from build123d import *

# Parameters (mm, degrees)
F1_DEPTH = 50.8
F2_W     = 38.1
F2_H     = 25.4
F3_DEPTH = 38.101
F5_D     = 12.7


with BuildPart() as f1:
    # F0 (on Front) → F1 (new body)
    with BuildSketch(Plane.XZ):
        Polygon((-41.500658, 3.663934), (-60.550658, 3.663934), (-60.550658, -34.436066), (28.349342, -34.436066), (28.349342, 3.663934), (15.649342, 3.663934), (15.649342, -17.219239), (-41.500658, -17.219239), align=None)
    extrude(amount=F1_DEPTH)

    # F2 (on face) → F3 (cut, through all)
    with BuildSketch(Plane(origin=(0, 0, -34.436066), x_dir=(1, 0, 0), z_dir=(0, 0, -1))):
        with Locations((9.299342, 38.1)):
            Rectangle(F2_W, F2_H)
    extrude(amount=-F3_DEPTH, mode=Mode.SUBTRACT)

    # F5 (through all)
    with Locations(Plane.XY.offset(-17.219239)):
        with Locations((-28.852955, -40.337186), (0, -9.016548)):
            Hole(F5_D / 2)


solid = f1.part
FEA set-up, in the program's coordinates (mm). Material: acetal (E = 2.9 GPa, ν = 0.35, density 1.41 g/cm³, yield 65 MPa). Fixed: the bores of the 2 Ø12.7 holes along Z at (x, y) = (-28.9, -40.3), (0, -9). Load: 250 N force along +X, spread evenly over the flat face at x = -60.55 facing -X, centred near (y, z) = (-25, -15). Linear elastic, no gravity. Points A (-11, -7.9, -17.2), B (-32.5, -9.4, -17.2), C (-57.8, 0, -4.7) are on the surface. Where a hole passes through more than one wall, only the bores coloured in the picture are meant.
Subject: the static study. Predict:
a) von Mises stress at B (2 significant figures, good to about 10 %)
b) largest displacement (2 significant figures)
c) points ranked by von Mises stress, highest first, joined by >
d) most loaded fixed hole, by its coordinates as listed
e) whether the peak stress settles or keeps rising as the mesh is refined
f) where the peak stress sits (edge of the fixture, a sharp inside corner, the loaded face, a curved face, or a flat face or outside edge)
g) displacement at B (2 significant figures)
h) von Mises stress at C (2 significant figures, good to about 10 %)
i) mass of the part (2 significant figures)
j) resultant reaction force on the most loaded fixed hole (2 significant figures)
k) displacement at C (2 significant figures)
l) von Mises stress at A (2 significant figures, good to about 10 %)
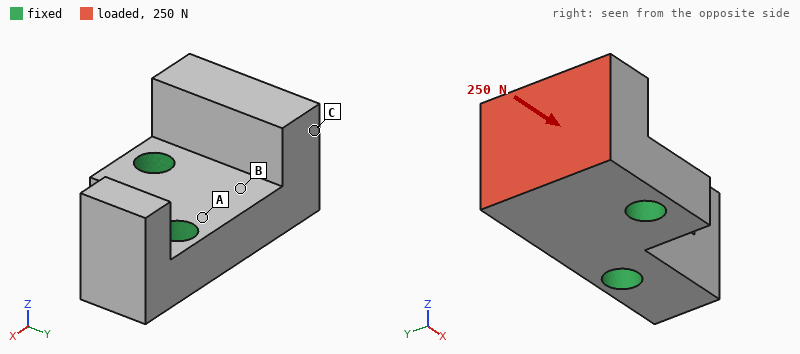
0.88 MPa
42 µm
B > A > C
(-28.9, -40.3)
keeps rising
edge of the fixture
6.9 µm
0.20 MPa
120 g
150 N
34 µm
0.57 MPa
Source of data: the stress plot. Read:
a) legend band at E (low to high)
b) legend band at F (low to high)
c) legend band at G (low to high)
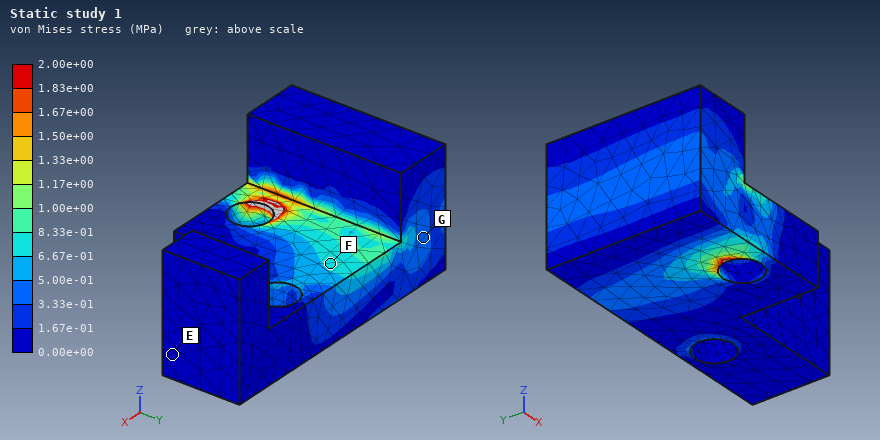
0.00e+00 to 1.67e-01 MPa
6.67e-01 to 8.33e-01 MPa
3.33e-01 to 5.00e-01 MPa
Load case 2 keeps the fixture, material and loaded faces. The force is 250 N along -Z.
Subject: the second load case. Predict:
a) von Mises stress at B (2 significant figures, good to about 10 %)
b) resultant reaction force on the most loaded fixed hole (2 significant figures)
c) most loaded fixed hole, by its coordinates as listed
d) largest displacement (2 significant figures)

1.3 MPa
260 N
(-28.9, -40.3)
0.11 mm
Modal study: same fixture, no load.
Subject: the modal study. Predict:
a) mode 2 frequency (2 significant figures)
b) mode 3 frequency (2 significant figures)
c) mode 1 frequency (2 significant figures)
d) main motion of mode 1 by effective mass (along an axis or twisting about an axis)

2300 Hz
2300 Hz
1500 Hz
along Z
